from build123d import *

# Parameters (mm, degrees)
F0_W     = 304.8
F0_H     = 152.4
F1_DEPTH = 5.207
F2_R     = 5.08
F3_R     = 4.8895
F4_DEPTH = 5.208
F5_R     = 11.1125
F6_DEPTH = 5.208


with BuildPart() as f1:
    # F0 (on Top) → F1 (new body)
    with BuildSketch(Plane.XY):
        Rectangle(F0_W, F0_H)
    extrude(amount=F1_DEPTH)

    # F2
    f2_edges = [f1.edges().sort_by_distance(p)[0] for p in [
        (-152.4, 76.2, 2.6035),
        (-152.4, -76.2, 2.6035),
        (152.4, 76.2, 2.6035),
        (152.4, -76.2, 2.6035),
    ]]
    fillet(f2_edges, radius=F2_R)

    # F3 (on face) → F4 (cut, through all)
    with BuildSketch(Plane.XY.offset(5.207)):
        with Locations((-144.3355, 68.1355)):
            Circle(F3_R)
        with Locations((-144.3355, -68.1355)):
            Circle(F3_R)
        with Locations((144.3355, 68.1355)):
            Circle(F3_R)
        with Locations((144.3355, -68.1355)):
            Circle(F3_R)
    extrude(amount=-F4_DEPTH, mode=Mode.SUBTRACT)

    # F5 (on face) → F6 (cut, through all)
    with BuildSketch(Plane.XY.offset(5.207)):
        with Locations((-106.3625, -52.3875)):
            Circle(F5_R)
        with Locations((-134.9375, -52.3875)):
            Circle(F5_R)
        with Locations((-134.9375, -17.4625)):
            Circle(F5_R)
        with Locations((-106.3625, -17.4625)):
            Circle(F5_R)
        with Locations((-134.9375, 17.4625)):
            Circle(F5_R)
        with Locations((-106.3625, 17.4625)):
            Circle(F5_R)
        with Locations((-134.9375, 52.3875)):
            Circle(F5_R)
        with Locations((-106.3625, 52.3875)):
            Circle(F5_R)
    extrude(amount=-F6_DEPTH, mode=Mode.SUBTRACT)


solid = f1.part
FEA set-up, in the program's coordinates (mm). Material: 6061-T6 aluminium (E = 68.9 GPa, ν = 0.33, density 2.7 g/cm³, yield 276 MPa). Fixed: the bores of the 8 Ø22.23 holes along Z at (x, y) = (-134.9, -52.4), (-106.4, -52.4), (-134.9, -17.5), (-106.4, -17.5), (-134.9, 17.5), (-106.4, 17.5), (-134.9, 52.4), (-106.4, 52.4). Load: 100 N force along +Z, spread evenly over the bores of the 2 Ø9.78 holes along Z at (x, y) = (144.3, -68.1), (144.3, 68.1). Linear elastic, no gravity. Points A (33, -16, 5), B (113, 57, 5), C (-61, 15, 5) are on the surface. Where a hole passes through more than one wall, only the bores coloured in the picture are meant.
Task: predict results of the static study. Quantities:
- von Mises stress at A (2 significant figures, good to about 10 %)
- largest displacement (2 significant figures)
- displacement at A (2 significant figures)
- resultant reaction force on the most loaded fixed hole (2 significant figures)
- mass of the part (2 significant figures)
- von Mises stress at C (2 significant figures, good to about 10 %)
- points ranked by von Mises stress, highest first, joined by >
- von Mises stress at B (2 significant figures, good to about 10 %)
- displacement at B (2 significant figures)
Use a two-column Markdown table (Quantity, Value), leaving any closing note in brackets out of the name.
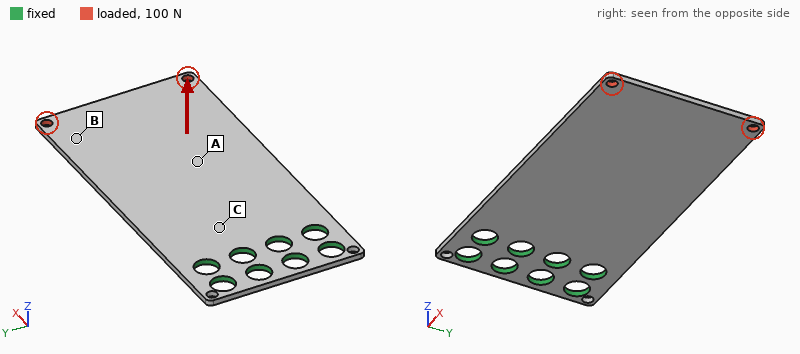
| Quantity | Value |
|---|---|
| von Mises stress at A | 15 MPa |
| largest displacement | 3.8 mm |
| displacement at A | 1.3 mm |
| resultant reaction force on the most loaded fixed hole | 60 N |
| mass of the part | 600 g |
| von Mises stress at C | 27 MPa |
| points ranked by von Mises stress, highest first, joined by > | C > A > B |
| von Mises stress at B | 6.1 MPa |
| displacement at B | 2.9 mm |
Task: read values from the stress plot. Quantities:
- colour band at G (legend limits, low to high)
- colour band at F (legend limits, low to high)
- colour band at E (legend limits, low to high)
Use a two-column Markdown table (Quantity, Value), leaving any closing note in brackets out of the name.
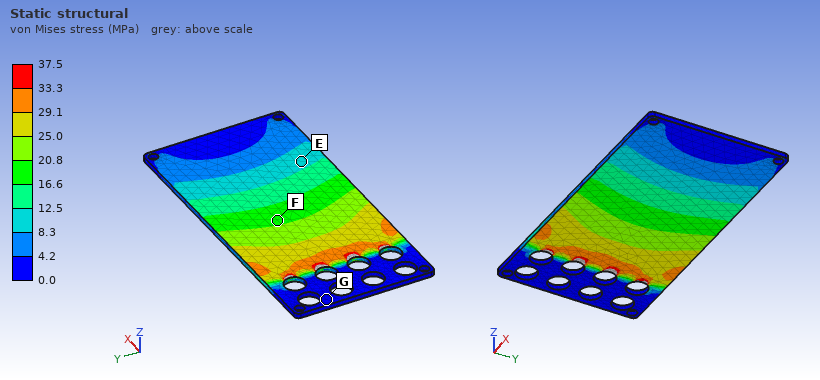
| Quantity | Value |
|---|---|
| colour band at G | 0.0 to 4.2 MPa |
| colour band at F | 16.6 to 20.8 MPa |
| colour band at E | 8.3 to 12.5 MPa |
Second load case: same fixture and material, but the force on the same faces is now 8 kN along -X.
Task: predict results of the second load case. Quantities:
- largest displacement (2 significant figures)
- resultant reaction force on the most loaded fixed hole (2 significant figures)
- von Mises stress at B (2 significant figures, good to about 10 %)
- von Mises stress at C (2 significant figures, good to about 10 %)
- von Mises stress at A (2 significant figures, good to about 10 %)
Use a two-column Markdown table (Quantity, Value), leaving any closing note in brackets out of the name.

| Quantity | Value |
|---|---|
| largest displacement | 72 µm |
| resultant reaction force on the most loaded fixed hole | 2.2 kN |
| von Mises stress at B | 19 MPa |
| von Mises stress at C | 10 MPa |
| von Mises stress at A | 8.6 MPa |
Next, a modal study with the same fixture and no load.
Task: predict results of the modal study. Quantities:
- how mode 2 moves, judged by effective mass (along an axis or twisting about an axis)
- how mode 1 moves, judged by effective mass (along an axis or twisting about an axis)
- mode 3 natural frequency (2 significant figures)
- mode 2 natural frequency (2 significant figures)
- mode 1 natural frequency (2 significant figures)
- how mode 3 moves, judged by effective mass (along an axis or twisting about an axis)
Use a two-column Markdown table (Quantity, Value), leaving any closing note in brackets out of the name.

| Quantity | Value |
|---|---|
| how mode 2 moves, judged by effective mass | twisting about X |
| how mode 1 moves, judged by effective mass | along Z |
| mode 3 natural frequency | 440 Hz |
| mode 2 natural frequency | 250 Hz |
| mode 1 natural frequency | 71 Hz |
| how mode 3 moves, judged by effective mass | along Z |
